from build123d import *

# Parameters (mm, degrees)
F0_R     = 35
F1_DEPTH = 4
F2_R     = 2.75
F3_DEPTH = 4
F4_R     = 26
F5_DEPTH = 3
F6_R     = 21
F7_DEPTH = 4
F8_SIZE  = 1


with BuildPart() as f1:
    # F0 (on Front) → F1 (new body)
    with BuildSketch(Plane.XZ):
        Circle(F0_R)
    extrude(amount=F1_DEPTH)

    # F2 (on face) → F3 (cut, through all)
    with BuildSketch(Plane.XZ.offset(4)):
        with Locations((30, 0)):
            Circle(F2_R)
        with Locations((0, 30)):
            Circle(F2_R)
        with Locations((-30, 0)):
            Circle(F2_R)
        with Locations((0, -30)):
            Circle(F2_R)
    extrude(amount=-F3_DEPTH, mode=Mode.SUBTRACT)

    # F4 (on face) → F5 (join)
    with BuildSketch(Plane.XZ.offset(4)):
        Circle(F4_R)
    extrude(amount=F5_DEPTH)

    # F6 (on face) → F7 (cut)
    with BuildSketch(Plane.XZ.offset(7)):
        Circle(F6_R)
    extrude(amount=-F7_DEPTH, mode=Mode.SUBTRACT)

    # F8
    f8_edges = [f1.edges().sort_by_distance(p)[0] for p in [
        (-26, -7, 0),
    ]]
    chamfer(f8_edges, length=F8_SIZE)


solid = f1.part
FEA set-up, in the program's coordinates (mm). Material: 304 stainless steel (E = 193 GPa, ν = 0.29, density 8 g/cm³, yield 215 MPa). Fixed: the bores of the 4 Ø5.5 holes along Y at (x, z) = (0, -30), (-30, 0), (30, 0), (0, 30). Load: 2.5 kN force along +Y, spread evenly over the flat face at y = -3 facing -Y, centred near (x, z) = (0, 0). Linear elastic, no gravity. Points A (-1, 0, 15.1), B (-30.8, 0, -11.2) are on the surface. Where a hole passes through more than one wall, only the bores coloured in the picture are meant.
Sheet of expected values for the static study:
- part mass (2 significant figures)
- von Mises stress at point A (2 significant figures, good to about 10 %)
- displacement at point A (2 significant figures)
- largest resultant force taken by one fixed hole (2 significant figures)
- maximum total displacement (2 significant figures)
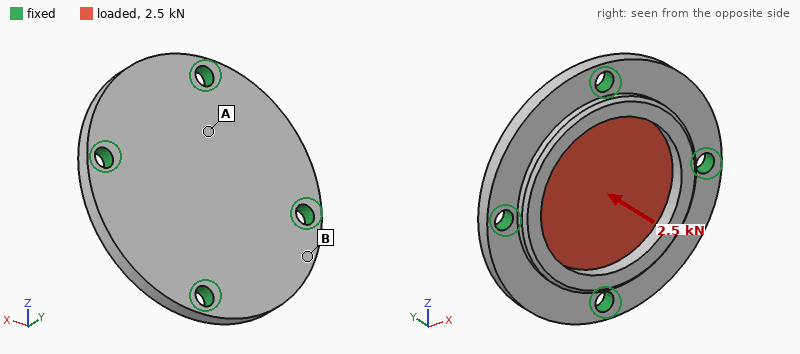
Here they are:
130 g
25 MPa
15 µm
630 N
30 µm
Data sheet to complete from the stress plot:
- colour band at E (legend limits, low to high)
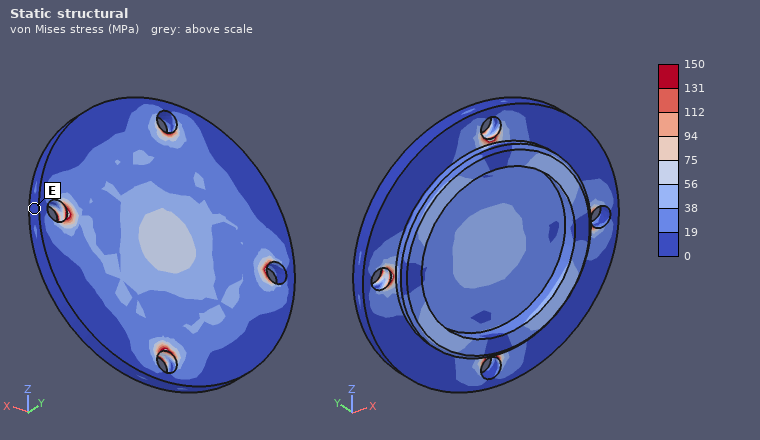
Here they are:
0 to 19 MPa
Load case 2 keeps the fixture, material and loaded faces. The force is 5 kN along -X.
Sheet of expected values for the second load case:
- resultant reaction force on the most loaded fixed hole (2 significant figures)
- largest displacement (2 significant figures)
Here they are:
1.5 kN
3.0 µm
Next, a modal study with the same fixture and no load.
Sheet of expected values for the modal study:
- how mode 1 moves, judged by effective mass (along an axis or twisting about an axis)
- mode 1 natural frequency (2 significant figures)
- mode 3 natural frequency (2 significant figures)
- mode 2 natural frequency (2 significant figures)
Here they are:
along Y
9300 Hz
12 kHz
11 kHz
